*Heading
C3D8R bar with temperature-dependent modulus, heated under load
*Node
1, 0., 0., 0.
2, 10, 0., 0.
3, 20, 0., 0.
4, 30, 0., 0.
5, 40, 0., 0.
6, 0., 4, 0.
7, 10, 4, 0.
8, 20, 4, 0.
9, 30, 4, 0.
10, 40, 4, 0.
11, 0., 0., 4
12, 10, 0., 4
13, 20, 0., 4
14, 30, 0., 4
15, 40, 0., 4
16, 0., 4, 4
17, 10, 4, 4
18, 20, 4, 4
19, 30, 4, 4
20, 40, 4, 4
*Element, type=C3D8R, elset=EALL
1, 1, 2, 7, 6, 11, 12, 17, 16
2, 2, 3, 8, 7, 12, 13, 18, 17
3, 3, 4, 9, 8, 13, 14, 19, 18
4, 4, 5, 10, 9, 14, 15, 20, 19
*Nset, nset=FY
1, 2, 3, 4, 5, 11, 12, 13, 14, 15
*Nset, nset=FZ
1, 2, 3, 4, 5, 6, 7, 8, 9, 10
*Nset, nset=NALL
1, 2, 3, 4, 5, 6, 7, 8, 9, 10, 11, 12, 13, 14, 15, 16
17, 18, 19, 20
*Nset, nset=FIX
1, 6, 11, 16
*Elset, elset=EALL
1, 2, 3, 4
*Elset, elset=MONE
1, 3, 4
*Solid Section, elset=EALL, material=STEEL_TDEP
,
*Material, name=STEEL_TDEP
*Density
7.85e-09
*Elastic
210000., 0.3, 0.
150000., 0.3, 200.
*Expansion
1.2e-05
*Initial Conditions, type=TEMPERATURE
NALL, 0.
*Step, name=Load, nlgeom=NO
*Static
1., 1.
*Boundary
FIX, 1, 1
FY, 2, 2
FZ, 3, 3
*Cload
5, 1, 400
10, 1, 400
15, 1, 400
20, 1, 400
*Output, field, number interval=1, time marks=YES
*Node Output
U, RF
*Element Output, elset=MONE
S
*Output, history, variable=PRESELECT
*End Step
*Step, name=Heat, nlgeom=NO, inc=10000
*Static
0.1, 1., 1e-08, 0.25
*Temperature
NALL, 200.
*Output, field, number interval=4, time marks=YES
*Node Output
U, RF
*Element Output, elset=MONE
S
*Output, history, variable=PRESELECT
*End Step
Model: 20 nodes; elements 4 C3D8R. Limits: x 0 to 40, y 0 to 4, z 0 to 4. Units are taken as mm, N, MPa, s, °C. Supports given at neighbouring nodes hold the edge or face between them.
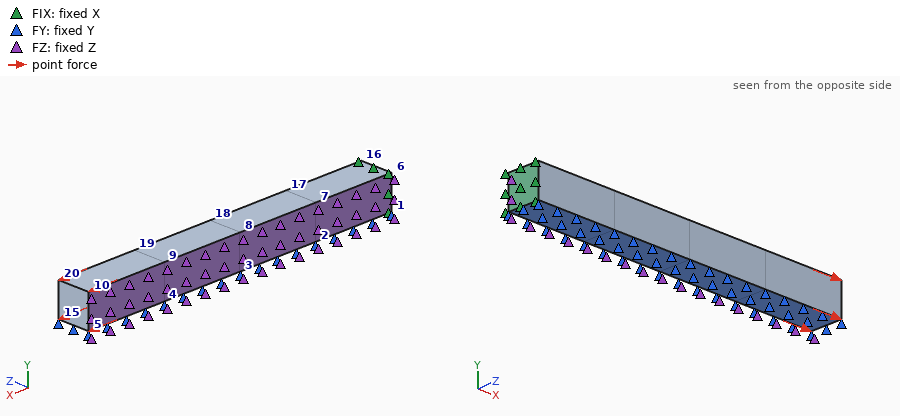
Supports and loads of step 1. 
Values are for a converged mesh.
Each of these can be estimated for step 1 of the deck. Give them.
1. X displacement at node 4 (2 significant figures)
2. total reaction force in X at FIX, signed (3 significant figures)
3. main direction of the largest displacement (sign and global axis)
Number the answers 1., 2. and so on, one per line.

1. 0.014 mm
2. -1600 N
3. +X
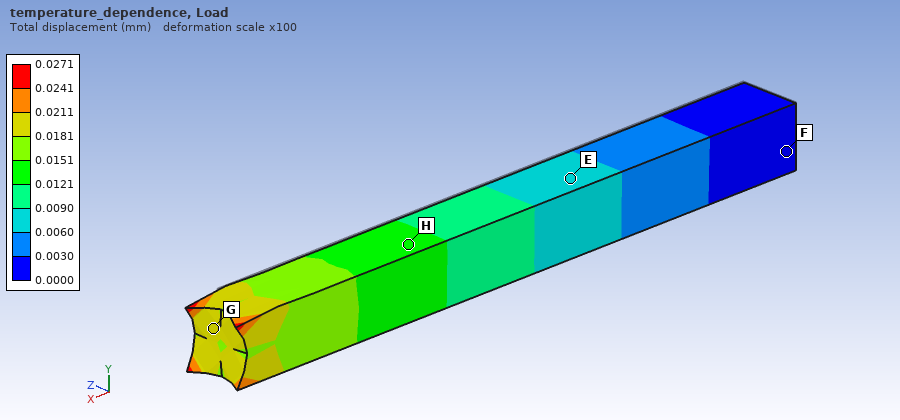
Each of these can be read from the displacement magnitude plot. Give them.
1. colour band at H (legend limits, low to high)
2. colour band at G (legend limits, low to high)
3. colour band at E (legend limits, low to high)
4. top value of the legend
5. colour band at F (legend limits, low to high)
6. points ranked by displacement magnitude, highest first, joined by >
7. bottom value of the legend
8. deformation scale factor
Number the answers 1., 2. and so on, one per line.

1. 0.0121 to 0.0151 mm
2. 0.0181 to 0.0211 mm
3. 0.0060 to 0.0090 mm
4. 0.0271 mm
5. 0.0000 to 0.0030 mm
6. G > H > E > F
7. 0.0000 mm
8. 100
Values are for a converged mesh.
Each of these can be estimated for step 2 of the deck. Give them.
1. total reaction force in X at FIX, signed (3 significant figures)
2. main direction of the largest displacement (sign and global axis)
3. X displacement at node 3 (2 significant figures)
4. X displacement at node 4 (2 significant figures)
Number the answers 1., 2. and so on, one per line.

1. -1600 N
2. +X
3. 0.061 mm
4. 0.092 mm
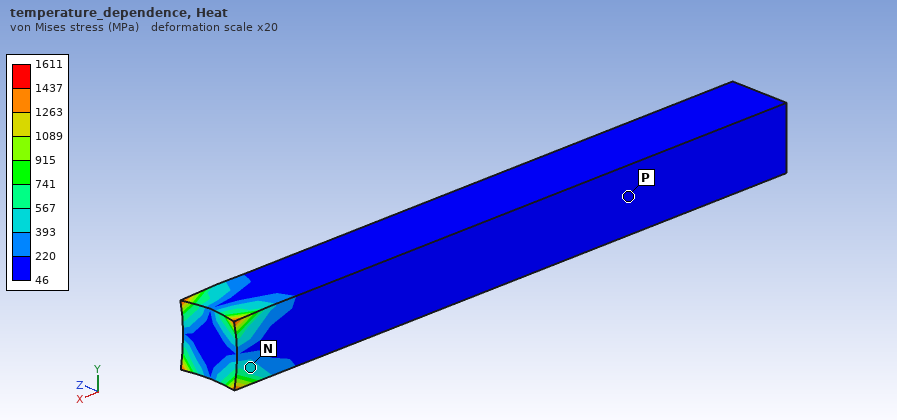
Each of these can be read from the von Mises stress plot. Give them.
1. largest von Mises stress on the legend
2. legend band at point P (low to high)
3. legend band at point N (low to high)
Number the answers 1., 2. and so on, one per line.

1. 1611 MPa
2. 46 to 220 MPa
3. 393 to 567 MPa
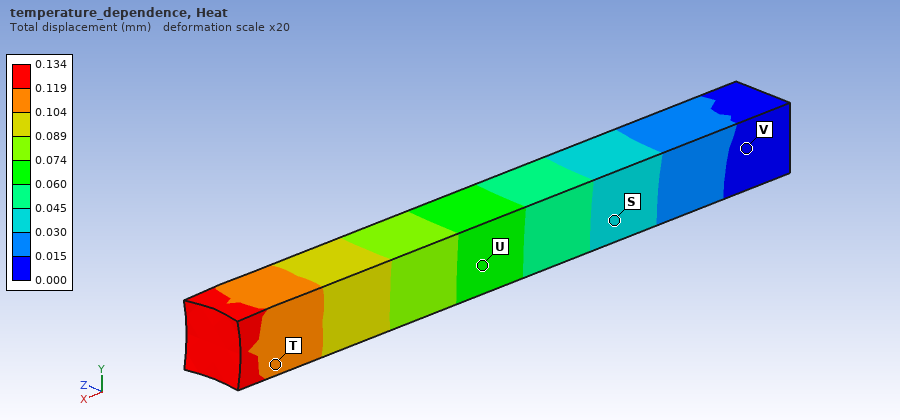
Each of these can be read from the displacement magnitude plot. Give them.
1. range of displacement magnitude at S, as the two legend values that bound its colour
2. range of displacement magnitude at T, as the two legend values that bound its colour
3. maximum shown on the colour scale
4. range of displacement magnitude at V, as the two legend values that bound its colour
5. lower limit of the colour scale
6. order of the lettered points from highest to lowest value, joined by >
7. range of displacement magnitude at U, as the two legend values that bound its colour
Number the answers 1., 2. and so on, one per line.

1. 0.030 to 0.045 mm
2. 0.104 to 0.119 mm
3. 0.134 mm
4. 0.000 to 0.015 mm
5. 0.000 mm
6. T > U > S > V
7. 0.060 to 0.074 mm
